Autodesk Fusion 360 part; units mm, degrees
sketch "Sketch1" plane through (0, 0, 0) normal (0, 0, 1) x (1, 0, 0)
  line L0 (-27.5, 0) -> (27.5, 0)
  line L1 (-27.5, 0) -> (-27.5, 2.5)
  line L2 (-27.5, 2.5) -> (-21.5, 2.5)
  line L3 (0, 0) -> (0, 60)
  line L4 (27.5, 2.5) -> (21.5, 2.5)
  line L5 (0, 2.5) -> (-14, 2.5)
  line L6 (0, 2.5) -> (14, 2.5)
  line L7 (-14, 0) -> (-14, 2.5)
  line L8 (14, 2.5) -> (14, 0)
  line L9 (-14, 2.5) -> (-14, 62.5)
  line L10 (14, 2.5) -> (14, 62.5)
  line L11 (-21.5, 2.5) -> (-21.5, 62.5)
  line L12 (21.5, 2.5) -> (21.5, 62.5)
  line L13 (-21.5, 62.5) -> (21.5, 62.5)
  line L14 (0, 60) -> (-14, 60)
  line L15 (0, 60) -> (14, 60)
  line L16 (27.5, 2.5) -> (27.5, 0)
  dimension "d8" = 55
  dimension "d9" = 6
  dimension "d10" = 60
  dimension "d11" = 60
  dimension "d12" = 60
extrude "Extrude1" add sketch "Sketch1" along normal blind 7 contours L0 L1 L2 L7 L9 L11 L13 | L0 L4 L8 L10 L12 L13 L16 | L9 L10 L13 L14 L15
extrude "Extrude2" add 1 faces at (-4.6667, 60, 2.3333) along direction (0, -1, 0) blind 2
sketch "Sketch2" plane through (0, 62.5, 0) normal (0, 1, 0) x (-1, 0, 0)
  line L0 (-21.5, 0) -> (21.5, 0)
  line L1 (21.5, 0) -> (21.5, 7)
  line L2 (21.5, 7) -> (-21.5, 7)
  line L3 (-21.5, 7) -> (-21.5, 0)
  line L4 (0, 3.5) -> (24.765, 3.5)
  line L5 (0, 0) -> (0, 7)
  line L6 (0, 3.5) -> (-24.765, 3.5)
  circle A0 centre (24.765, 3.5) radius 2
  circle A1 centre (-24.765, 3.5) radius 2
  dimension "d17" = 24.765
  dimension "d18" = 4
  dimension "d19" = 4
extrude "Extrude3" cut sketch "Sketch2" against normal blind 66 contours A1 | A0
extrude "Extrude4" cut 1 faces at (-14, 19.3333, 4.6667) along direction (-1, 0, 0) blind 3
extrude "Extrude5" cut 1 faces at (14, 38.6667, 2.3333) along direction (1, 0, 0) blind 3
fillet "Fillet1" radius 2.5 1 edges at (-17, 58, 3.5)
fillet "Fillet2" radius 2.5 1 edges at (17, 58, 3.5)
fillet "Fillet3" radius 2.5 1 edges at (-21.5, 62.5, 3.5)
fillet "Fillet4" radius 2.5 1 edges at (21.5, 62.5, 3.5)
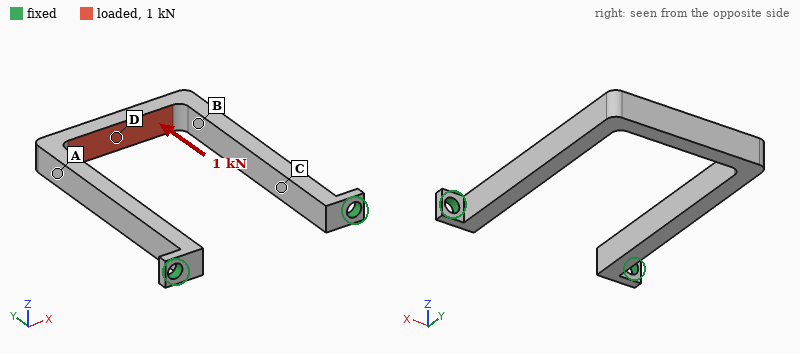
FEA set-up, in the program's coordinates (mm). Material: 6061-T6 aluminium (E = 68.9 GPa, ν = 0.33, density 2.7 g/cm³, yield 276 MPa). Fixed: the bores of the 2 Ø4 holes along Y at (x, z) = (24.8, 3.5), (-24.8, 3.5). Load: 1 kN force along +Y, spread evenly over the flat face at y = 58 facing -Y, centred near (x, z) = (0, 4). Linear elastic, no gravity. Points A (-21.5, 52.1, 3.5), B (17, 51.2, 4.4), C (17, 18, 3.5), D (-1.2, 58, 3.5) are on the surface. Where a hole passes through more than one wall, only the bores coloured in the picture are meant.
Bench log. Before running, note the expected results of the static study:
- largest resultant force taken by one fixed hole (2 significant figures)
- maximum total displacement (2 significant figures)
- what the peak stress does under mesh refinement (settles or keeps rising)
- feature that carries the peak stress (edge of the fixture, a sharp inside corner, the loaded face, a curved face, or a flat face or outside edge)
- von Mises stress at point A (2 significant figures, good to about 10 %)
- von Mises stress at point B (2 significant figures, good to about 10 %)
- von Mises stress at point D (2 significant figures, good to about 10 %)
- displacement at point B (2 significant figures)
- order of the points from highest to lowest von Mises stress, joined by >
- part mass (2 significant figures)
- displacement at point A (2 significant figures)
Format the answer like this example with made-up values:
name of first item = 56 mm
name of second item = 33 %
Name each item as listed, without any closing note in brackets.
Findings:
largest resultant force taken by one fixed hole = 500 N
maximum total displacement = 0.15 mm
what the peak stress does under mesh refinement = keeps rising
feature that carries the peak stress = edge of the fixture
von Mises stress at point A = 67 MPa
von Mises stress at point B = 96 MPa
von Mises stress at point D = 140 MPa
displacement at point B = 0.067 mm
order of the points from highest to lowest von Mises stress, joined by > = D > B > A > C
part mass = 14 g
displacement at point A = 0.058 mm
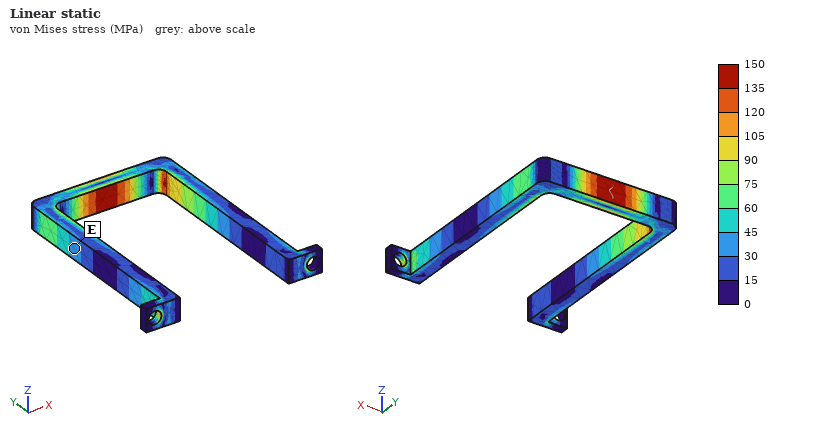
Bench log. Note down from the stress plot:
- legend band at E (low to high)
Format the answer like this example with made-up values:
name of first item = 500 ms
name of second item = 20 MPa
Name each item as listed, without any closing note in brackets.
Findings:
legend band at E = 30 to 45 MPa
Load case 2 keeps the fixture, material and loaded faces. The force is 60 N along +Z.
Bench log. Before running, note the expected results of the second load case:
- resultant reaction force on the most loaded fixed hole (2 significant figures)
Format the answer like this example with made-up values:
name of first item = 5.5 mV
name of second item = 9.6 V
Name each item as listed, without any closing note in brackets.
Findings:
resultant reaction force on the most loaded fixed hole = 30 N
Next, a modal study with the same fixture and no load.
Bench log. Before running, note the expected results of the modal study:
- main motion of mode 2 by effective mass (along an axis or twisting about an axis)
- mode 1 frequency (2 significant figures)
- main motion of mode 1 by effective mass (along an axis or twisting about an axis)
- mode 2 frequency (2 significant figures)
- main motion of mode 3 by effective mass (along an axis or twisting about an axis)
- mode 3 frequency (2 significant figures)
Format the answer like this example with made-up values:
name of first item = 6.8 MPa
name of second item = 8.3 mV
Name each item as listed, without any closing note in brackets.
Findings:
main motion of mode 2 by effective mass = along X
mode 1 frequency = 720 Hz
main motion of mode 1 by effective mass = along Z
mode 2 frequency = 930 Hz
main motion of mode 3 by effective mass = twisting about Y
mode 3 frequency = 1700 Hz
